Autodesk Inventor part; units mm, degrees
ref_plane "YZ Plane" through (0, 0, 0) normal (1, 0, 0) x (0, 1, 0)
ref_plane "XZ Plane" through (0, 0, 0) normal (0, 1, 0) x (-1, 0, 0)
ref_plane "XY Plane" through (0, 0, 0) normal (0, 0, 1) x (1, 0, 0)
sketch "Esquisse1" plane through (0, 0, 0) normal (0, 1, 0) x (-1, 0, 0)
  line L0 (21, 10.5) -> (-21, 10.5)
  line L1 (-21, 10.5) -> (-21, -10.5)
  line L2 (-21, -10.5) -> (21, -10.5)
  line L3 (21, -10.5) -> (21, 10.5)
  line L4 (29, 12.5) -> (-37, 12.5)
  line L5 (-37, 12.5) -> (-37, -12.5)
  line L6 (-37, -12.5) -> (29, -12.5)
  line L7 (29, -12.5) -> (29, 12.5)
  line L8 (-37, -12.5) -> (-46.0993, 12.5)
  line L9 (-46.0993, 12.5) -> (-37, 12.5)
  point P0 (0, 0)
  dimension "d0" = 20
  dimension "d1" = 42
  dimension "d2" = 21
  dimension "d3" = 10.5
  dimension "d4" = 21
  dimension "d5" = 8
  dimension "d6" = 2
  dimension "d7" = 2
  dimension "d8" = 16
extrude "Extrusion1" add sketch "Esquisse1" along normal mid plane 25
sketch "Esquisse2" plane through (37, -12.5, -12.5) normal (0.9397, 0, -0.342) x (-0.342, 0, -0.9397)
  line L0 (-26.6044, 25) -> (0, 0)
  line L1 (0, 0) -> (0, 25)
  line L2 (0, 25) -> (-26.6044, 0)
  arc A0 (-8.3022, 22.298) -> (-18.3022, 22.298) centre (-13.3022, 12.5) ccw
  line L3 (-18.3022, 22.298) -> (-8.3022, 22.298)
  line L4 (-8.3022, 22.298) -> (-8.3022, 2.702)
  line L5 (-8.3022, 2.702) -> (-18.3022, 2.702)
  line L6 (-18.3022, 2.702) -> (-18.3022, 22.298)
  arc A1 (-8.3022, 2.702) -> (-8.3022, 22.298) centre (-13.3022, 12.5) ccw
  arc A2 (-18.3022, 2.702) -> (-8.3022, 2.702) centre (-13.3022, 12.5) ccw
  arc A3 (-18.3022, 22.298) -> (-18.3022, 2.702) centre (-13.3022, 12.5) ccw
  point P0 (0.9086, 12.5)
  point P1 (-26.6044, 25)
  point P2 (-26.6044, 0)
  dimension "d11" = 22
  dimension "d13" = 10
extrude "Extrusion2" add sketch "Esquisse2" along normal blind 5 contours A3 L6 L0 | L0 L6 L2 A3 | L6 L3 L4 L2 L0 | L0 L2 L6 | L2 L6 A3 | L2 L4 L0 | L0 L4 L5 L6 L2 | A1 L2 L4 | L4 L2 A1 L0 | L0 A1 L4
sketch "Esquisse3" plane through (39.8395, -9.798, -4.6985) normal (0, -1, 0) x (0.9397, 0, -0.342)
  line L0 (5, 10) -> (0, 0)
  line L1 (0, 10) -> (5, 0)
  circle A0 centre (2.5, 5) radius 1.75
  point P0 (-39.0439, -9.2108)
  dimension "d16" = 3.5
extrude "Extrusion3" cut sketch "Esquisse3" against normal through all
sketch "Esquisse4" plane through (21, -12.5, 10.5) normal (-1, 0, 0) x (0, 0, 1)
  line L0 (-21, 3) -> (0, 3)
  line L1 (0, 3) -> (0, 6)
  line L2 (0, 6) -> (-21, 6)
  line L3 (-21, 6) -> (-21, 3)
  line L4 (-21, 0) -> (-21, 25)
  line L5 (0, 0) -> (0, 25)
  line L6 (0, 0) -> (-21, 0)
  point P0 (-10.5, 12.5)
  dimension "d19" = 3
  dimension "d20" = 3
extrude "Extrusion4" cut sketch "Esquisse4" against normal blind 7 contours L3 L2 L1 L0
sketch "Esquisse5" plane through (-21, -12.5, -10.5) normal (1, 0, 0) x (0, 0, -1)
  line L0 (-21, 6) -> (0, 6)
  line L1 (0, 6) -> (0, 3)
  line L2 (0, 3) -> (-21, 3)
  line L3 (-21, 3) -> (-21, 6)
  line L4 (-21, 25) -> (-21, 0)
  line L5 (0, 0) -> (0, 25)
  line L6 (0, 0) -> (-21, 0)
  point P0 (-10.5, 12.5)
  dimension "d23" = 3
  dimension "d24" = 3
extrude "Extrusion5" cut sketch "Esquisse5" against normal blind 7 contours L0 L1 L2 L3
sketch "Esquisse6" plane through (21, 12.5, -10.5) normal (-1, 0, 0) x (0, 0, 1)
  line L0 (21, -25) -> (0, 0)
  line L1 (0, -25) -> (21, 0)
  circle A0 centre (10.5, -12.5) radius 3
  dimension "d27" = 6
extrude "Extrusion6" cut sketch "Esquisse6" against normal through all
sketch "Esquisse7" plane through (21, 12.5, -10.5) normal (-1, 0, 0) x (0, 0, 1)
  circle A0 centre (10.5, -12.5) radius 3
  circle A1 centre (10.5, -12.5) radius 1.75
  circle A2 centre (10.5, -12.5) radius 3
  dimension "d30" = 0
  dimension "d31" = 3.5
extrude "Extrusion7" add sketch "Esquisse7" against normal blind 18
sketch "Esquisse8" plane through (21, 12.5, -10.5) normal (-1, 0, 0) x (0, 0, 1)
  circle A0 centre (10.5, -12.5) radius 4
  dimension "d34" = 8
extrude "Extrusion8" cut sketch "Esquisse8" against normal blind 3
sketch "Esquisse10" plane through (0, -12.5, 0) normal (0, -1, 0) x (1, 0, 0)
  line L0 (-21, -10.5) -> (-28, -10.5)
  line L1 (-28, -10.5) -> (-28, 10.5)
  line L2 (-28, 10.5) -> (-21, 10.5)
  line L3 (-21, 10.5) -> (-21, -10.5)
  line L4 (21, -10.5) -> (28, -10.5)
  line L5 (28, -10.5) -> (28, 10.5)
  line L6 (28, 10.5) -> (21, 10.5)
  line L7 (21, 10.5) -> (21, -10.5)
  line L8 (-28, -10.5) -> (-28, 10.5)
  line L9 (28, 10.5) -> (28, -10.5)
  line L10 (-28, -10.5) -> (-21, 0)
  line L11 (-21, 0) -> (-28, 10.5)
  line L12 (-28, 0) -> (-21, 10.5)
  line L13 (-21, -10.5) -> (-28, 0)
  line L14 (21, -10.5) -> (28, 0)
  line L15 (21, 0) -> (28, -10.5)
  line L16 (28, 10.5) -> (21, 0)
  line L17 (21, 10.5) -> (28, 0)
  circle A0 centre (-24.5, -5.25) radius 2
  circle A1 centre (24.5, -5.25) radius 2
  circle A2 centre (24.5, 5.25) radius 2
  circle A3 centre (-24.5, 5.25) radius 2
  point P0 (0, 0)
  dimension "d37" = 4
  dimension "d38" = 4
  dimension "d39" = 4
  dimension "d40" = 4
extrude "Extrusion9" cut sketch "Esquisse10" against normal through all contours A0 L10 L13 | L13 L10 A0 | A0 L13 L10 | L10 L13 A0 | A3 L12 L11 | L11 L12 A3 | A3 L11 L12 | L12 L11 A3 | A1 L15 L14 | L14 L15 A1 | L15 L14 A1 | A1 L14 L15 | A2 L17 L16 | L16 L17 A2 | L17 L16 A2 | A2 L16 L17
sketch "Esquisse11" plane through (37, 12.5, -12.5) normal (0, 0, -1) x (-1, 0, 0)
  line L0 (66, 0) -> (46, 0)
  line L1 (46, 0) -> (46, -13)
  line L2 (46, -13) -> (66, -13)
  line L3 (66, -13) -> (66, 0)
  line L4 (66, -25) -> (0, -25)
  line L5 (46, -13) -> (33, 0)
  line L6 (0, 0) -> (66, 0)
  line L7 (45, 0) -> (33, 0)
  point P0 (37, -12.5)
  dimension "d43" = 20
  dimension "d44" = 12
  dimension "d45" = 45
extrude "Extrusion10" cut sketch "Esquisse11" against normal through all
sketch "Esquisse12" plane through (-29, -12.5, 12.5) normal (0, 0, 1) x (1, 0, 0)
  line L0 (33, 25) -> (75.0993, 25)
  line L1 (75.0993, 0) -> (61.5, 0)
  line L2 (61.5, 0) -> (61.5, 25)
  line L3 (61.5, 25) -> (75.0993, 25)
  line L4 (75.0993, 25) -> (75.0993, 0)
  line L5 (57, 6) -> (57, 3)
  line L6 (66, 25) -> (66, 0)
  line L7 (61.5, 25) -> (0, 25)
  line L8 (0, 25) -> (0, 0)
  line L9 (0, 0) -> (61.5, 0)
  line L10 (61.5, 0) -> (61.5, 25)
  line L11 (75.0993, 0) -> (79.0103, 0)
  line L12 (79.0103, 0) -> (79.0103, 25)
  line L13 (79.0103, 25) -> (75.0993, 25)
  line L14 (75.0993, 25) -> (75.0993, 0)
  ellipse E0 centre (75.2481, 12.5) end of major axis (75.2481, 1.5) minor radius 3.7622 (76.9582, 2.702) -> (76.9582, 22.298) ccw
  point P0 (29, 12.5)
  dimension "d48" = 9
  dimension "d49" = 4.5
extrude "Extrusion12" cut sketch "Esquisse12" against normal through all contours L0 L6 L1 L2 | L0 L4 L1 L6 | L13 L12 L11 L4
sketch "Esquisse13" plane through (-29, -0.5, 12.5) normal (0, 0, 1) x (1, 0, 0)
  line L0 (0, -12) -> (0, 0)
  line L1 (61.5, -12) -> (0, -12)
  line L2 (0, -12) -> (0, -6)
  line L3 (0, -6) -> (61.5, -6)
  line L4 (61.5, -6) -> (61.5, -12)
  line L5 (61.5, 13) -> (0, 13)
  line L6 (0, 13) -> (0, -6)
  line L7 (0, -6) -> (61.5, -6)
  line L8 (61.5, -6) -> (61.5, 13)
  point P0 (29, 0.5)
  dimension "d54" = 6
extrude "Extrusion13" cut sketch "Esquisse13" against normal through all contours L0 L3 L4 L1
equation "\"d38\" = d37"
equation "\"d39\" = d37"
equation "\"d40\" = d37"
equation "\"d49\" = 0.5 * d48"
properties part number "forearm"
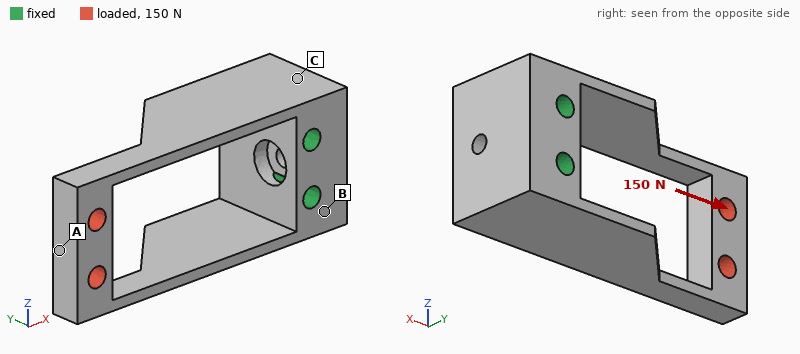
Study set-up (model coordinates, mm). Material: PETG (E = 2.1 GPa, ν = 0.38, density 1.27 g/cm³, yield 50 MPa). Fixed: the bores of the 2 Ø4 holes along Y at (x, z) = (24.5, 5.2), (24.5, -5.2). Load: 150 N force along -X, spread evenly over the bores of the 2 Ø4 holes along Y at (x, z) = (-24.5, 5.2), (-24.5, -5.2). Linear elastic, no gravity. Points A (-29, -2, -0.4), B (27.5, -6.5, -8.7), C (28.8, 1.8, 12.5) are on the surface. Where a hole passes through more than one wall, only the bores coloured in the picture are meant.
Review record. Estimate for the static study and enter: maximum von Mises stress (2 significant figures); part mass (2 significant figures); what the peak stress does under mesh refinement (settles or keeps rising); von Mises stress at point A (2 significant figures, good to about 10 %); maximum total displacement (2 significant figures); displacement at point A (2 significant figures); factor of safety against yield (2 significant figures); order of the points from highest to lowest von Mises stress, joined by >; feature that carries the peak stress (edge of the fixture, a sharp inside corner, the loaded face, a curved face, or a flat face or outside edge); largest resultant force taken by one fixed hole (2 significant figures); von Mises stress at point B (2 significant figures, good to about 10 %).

11 MPa
10 g
settles
8.7 MPa
0.41 mm
0.38 mm
4.4
A > B > C
a flat face or outside edge
81 N
2.0 MPa
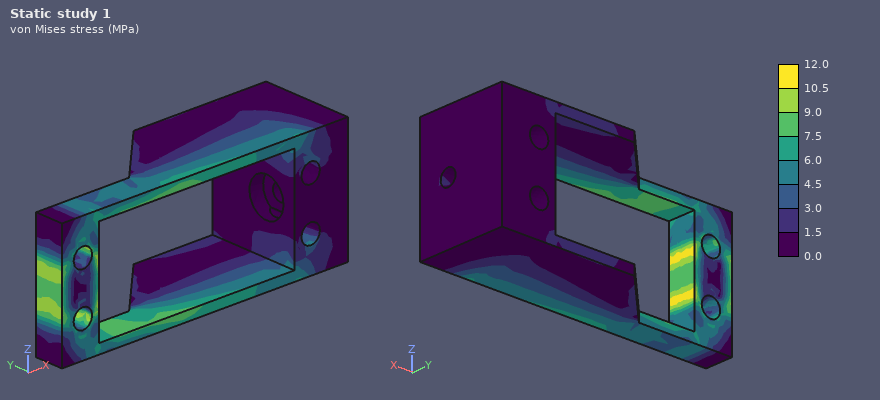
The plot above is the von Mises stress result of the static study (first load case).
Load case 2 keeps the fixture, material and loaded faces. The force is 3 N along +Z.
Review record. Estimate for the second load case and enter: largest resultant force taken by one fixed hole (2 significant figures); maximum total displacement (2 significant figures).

6.7 N
0.68 mm
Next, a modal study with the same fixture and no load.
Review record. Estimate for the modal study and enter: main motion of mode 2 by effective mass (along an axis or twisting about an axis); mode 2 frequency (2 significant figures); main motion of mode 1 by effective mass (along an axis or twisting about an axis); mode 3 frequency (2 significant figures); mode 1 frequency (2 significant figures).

along Y
760 Hz
along Z
1200 Hz
250 Hz
